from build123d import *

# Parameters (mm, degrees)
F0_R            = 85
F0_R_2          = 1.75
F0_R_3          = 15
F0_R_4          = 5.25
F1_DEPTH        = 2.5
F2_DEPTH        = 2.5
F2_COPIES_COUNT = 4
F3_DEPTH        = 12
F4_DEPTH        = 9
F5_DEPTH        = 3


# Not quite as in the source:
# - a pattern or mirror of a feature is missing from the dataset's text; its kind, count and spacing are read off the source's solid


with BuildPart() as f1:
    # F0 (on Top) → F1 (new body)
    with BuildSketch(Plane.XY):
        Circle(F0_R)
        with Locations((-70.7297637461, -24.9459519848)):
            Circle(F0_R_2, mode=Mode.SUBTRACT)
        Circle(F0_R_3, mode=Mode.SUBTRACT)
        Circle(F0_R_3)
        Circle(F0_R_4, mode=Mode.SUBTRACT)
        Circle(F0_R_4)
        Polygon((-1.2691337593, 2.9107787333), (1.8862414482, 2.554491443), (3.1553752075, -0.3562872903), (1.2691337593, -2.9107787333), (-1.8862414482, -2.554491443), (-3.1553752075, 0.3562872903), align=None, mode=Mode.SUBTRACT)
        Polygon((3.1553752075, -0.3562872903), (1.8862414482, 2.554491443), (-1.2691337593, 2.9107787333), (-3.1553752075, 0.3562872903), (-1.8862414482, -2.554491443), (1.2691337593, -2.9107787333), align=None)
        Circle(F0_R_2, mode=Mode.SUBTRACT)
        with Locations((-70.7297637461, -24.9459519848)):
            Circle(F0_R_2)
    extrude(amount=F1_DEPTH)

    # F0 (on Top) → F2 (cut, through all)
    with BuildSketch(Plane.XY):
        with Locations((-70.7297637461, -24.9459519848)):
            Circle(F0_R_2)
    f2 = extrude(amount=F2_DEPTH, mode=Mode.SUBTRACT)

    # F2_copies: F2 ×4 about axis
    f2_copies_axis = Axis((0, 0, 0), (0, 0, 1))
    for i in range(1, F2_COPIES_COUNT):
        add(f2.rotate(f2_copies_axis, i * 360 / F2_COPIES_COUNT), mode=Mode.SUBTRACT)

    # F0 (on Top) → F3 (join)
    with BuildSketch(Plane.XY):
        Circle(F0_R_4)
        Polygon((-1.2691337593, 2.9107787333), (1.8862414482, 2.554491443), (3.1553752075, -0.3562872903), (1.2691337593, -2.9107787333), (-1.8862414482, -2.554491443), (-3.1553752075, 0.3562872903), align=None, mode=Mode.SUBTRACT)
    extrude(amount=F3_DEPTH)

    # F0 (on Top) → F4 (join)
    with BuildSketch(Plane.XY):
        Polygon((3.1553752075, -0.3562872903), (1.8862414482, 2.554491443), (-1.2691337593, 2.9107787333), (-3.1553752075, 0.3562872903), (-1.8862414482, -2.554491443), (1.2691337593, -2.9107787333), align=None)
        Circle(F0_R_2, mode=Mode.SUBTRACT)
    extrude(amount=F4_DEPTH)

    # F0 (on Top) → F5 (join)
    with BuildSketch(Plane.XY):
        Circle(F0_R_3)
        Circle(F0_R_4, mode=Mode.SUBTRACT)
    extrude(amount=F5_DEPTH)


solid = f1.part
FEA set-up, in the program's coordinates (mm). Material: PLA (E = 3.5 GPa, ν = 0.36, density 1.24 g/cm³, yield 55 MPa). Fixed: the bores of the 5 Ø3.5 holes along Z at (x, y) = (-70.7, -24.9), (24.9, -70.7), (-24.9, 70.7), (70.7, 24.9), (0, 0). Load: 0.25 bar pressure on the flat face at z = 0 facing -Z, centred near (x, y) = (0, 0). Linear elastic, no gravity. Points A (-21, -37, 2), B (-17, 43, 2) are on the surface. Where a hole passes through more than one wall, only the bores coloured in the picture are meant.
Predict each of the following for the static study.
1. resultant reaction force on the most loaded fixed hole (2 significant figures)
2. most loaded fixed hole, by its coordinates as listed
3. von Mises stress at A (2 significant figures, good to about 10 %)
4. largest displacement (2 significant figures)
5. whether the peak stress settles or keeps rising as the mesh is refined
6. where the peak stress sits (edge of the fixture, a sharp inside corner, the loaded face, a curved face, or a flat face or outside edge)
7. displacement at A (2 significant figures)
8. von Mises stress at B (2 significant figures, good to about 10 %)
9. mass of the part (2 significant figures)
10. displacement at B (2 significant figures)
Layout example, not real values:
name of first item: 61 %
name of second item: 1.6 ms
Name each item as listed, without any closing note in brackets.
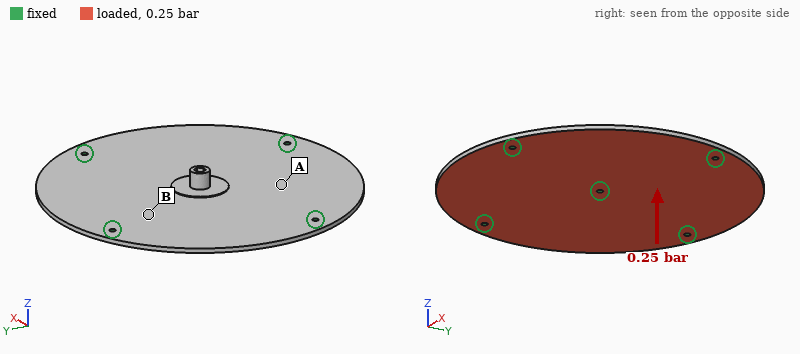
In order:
resultant reaction force on the most loaded fixed hole: 160 N
most loaded fixed hole, by its coordinates as listed: (0, 0)
von Mises stress at A: 4.2 MPa
largest displacement: 2.8 mm
whether the peak stress settles or keeps rising as the mesh is refined: keeps rising
where the peak stress sits: edge of the fixture
displacement at A: 1.0 mm
von Mises stress at B: 11 MPa
mass of the part: 71 g
displacement at B: 0.61 mm
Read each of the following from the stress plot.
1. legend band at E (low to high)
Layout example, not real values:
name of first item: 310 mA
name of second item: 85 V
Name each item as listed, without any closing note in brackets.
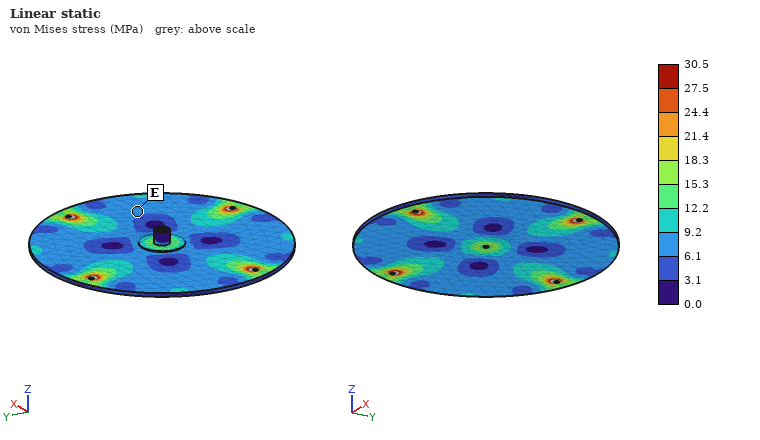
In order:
legend band at E: 6.1 to 9.2 MPa
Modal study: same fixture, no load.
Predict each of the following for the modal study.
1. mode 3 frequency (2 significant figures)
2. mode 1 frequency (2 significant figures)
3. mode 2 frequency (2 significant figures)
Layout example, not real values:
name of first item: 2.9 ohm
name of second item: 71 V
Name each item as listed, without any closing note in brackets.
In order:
mode 3 frequency: 330 Hz
mode 1 frequency: 300 Hz
mode 2 frequency: 330 Hz
